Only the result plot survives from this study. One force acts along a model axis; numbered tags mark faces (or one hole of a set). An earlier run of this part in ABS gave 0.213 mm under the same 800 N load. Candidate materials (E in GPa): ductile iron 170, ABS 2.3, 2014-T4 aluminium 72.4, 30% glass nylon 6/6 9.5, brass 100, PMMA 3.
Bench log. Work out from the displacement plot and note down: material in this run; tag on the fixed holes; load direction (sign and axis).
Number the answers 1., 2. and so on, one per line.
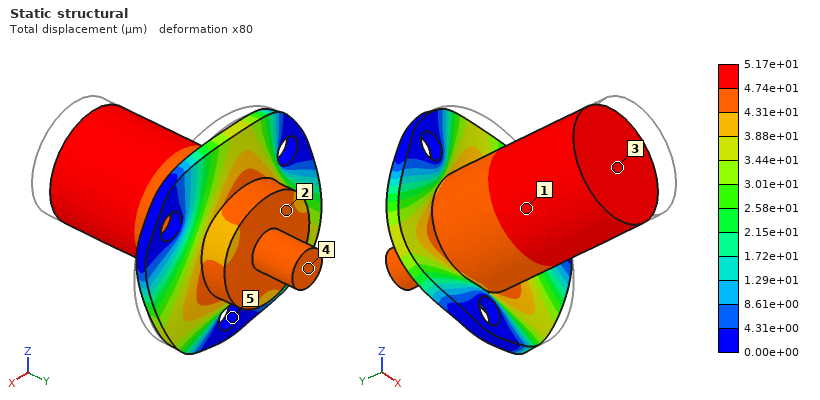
1. 30% glass nylon 6/6
2. 5
3. +Y
